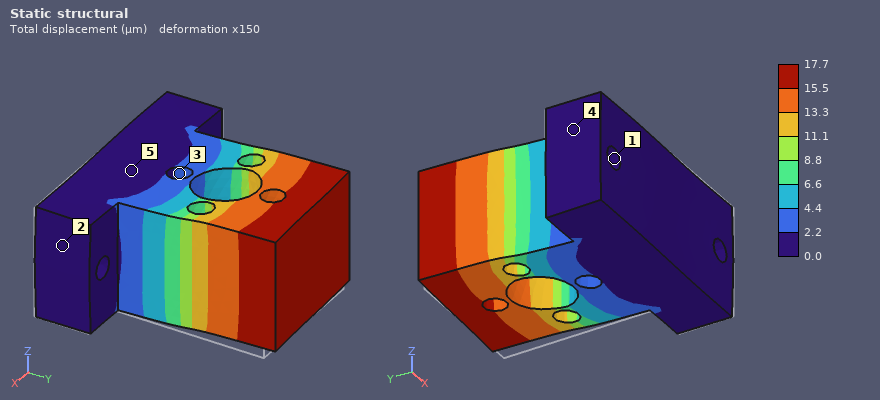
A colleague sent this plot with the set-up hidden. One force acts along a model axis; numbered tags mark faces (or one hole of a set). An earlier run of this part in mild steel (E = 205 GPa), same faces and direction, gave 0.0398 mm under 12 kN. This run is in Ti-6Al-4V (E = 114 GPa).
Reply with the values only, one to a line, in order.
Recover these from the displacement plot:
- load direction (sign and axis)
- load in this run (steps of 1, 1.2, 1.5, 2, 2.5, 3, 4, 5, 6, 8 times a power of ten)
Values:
-X
3 kN
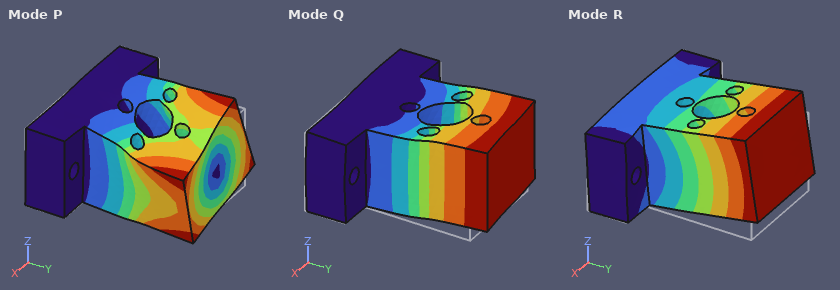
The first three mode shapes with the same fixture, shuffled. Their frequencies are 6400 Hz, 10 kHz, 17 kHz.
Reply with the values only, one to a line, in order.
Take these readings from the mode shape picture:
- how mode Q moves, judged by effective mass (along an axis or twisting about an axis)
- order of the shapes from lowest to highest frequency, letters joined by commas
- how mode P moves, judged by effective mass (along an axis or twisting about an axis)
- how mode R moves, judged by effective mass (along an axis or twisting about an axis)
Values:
along X
R, Q, P
twisting about Y
along Z
